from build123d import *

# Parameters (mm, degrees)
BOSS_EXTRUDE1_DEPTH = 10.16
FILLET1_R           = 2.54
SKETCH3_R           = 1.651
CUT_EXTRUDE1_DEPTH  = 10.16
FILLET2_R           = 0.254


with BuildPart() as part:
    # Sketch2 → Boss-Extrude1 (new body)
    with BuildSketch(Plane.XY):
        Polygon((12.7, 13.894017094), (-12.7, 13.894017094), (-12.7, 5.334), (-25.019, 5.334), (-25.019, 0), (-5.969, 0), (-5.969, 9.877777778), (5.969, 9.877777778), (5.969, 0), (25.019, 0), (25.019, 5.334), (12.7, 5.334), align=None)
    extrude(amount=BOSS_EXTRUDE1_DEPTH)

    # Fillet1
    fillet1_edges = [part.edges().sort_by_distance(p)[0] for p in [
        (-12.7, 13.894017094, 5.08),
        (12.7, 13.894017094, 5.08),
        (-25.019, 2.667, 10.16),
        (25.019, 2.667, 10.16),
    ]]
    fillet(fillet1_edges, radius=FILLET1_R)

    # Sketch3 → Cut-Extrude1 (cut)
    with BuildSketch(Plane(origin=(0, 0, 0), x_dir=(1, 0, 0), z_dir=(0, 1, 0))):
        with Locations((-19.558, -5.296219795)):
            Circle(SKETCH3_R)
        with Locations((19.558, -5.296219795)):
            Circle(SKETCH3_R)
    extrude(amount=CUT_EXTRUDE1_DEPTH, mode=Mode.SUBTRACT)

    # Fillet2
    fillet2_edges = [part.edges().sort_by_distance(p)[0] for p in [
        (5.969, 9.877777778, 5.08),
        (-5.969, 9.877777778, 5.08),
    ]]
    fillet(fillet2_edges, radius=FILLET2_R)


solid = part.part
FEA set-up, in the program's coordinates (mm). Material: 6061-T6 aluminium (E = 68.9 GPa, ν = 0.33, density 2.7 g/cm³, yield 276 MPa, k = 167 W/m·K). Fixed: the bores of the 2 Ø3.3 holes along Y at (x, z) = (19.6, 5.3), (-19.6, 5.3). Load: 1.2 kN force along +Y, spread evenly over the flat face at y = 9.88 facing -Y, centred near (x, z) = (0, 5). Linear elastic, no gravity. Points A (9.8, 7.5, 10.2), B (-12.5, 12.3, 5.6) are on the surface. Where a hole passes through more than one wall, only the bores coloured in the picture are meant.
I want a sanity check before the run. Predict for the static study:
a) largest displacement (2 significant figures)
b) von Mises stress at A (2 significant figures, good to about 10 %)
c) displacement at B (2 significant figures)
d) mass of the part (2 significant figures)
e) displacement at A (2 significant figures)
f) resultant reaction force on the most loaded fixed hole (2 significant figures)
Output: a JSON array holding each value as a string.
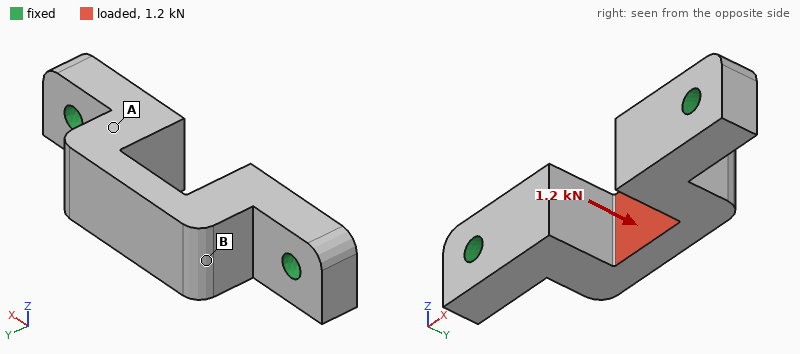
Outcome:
["19 µm", "26 MPa", "8.5 µm", "9.7 g", "9.2 µm", "860 N"]
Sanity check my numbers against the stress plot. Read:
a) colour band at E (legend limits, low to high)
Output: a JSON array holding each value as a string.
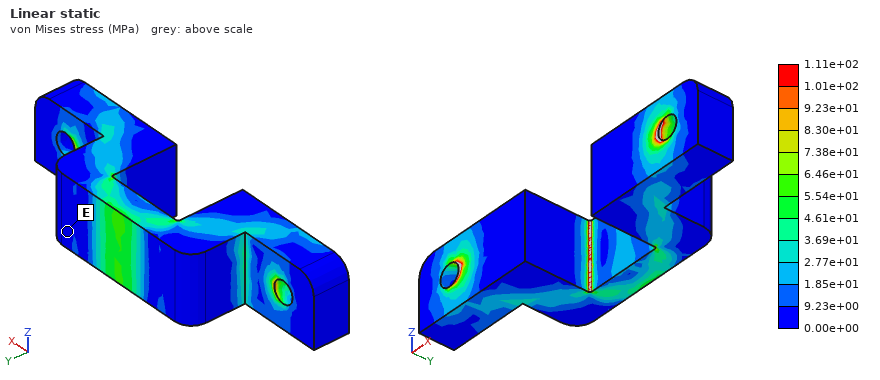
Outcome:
["0.00e+00 to 9.23e+00 MPa"]
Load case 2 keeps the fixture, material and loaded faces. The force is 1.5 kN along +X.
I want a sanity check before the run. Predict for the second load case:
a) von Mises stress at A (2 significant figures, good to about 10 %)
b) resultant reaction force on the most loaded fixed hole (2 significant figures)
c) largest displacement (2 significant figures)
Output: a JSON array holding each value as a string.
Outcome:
["33 MPa", "790 N", "23 µm"]
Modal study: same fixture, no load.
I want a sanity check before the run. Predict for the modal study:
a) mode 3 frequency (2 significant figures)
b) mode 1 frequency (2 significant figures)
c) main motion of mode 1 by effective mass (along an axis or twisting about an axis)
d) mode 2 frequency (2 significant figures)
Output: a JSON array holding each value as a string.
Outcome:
["22 kHz", "11 kHz", "along Z", "21 kHz"]
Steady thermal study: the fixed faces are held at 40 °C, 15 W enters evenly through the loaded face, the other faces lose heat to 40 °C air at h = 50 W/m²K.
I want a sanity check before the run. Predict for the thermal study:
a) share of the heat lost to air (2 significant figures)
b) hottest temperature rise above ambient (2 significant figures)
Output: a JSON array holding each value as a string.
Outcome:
["4.4 %", "17 K"]
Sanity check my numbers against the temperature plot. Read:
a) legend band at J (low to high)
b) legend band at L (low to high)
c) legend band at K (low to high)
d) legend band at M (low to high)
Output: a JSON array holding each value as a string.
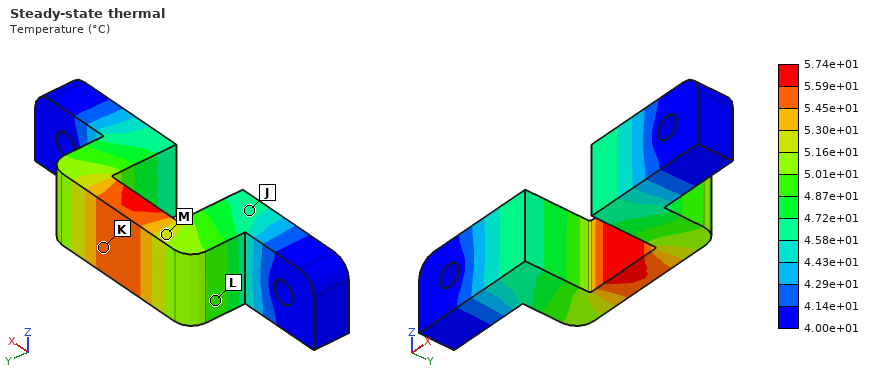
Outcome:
["4.58e+01 to 4.72e+01 °C", "4.87e+01 to 5.01e+01 °C", "5.45e+01 to 5.59e+01 °C", "5.16e+01 to 5.30e+01 °C"]
